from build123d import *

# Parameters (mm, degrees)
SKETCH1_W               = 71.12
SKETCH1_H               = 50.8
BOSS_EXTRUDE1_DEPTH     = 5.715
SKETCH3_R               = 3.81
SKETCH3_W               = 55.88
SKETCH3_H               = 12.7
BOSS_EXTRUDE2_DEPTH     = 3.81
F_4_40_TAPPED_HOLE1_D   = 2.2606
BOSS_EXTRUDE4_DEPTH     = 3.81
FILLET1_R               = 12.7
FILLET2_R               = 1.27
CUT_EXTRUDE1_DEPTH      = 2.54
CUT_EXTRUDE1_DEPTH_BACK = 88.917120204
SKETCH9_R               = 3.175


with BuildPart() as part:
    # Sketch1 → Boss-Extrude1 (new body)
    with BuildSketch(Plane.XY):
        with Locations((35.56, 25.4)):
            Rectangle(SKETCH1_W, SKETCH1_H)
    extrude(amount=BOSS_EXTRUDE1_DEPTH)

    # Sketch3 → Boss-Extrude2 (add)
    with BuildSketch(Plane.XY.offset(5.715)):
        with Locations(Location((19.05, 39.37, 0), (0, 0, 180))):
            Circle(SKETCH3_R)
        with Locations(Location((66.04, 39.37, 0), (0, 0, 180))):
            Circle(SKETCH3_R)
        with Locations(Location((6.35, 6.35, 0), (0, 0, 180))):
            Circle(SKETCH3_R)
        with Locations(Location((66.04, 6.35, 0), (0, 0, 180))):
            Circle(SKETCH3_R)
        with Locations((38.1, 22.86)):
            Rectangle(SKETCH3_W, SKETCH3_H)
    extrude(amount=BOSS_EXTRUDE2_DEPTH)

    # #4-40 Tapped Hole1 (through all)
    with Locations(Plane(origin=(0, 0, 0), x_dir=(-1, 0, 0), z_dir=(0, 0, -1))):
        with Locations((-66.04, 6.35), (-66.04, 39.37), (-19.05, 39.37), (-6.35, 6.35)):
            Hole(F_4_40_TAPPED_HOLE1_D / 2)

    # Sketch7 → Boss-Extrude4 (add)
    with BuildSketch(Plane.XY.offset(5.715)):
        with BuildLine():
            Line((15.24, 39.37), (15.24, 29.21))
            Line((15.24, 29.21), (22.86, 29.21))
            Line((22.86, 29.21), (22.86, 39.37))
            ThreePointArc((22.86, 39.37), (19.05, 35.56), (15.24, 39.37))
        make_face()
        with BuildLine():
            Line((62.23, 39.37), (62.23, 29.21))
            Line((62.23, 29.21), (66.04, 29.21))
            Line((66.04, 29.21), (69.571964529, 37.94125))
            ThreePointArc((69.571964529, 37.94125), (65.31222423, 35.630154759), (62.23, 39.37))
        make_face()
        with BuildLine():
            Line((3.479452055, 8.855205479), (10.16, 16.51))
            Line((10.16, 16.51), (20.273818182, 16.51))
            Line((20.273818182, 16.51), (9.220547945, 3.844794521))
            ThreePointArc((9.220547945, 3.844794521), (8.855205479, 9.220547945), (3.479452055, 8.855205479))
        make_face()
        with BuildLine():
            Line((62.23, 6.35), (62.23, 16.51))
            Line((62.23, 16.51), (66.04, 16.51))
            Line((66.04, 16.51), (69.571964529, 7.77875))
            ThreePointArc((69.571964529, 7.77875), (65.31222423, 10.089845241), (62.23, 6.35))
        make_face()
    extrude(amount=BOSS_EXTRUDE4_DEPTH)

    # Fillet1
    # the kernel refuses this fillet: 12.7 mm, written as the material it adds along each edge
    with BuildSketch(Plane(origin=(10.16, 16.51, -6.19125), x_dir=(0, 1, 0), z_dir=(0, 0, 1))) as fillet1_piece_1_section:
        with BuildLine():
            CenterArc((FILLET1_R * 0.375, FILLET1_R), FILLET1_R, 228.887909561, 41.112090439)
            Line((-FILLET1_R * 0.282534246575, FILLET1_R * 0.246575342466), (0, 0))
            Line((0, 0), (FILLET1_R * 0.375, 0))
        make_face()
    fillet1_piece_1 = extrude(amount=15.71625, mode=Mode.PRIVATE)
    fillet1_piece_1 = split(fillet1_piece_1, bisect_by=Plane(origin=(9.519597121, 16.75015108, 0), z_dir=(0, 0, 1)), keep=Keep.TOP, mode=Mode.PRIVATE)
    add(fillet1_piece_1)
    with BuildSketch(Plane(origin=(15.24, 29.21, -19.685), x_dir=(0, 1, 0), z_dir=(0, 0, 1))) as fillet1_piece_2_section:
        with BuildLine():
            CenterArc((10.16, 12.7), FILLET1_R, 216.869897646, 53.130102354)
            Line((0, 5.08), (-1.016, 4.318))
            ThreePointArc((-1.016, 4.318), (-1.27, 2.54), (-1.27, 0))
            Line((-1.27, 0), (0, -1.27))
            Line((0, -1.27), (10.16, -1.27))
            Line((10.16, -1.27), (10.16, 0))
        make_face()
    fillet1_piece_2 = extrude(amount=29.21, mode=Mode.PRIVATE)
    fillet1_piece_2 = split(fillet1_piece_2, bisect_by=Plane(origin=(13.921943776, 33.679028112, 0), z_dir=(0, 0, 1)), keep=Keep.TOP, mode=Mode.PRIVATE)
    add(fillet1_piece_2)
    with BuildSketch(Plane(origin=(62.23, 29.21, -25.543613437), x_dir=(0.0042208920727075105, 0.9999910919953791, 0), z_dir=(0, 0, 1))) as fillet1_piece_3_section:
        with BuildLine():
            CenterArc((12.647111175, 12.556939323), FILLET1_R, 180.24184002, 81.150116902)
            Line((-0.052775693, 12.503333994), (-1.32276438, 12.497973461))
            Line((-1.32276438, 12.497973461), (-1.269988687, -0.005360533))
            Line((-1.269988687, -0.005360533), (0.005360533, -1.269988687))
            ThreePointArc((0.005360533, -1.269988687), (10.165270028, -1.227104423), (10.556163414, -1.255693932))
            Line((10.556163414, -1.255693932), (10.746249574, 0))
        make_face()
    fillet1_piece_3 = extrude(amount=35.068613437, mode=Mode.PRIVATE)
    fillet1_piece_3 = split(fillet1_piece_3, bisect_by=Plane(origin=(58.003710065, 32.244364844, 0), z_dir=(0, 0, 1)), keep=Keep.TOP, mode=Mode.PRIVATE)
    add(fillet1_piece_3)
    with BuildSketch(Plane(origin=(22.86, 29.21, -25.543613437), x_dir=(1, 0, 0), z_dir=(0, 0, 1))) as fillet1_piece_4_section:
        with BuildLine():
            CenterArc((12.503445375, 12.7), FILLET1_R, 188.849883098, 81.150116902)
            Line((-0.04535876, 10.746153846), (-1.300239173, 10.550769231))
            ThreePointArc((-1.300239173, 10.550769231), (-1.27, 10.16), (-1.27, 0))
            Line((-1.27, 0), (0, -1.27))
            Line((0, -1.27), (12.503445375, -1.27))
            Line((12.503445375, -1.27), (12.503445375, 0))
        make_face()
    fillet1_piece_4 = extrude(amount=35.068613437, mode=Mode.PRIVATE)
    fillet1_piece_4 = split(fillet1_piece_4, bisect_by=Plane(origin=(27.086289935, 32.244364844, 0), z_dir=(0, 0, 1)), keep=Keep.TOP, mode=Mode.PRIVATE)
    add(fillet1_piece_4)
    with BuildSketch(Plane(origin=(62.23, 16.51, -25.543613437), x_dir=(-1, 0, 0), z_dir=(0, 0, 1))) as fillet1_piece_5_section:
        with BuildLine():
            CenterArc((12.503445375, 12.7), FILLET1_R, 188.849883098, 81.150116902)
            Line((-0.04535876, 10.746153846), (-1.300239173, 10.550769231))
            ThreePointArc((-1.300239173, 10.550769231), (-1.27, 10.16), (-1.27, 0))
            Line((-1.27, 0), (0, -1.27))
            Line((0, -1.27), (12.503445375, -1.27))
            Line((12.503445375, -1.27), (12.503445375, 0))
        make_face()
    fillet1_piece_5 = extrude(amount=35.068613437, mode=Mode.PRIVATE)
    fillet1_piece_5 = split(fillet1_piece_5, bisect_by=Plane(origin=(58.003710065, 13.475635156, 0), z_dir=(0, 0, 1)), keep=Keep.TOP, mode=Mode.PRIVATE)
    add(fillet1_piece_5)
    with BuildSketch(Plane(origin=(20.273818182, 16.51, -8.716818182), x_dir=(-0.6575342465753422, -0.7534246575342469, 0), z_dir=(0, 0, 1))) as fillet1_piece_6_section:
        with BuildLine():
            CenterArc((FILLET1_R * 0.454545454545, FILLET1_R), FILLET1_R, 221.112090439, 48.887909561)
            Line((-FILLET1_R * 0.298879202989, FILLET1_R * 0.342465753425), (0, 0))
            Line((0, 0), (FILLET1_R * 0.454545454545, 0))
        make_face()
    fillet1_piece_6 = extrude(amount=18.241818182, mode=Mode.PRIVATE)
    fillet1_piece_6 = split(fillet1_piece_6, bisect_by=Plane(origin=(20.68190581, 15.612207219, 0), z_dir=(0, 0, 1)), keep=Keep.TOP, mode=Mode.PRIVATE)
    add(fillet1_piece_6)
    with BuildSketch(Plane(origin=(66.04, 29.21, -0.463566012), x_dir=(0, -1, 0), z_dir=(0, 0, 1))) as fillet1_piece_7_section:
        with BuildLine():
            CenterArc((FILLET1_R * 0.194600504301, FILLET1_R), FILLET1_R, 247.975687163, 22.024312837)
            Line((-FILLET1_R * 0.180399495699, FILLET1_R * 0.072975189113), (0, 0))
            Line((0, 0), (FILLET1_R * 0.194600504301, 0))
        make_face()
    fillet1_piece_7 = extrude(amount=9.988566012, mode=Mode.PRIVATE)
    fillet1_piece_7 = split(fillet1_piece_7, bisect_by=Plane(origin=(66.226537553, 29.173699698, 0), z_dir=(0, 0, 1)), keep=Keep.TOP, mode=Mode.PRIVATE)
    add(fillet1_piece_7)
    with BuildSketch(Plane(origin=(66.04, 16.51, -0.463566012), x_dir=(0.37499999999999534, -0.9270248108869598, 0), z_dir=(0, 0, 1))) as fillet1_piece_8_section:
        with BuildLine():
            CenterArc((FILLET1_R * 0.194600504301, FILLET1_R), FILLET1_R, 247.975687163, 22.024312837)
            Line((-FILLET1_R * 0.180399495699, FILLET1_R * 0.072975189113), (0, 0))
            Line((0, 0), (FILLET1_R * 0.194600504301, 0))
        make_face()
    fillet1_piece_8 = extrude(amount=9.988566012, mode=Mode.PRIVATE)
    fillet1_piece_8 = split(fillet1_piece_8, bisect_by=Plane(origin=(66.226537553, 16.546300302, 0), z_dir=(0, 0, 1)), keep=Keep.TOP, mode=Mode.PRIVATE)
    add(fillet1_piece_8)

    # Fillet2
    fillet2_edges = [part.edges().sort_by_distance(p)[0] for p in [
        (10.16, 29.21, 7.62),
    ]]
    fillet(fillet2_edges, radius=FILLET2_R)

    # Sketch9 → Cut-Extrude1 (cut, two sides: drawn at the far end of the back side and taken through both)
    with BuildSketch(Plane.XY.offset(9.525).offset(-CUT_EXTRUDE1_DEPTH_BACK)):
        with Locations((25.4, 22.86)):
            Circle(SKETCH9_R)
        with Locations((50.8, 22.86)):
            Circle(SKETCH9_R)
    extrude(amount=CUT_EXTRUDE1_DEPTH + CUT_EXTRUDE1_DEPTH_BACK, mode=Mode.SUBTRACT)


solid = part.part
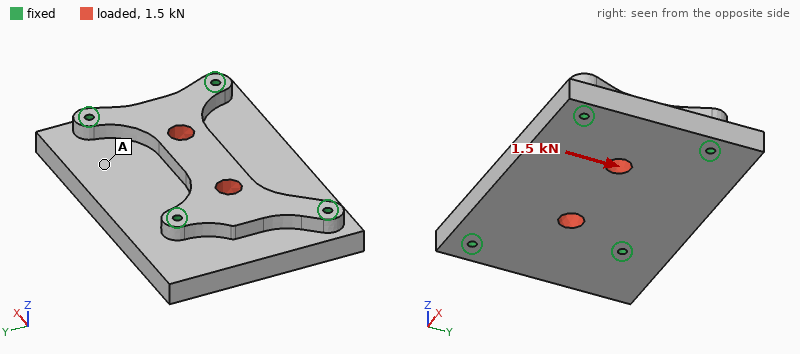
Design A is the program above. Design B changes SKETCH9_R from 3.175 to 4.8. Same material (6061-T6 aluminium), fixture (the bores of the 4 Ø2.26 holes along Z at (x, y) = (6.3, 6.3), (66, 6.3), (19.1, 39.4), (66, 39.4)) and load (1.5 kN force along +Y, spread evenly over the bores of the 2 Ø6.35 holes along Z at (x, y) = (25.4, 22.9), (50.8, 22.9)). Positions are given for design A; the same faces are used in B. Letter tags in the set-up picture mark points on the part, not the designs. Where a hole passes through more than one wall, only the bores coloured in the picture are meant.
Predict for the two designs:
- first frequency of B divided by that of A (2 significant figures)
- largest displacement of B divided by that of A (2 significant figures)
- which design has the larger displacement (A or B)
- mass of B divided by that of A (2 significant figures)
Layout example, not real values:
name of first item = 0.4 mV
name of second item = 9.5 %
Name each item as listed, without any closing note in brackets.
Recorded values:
first frequency of B divided by that of A = 0.99
largest displacement of B divided by that of A = 1.2
which design has the larger displacement = B
mass of B divided by that of A = 0.97
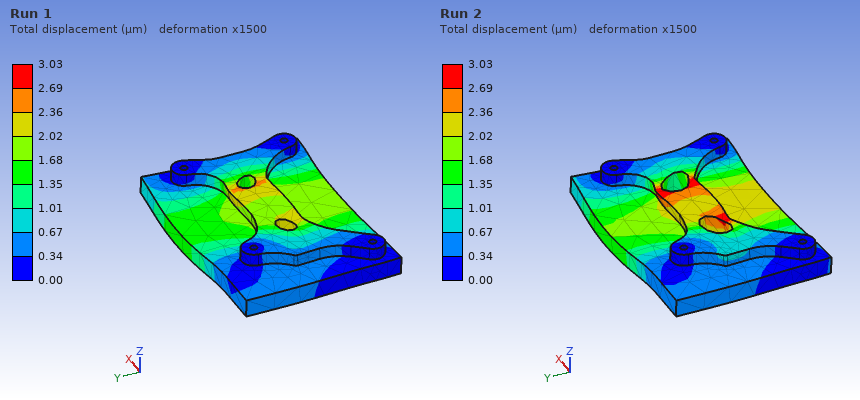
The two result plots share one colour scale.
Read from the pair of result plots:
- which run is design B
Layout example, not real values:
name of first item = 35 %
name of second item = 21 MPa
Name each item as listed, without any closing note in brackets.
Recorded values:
which run is design B = Run 2
